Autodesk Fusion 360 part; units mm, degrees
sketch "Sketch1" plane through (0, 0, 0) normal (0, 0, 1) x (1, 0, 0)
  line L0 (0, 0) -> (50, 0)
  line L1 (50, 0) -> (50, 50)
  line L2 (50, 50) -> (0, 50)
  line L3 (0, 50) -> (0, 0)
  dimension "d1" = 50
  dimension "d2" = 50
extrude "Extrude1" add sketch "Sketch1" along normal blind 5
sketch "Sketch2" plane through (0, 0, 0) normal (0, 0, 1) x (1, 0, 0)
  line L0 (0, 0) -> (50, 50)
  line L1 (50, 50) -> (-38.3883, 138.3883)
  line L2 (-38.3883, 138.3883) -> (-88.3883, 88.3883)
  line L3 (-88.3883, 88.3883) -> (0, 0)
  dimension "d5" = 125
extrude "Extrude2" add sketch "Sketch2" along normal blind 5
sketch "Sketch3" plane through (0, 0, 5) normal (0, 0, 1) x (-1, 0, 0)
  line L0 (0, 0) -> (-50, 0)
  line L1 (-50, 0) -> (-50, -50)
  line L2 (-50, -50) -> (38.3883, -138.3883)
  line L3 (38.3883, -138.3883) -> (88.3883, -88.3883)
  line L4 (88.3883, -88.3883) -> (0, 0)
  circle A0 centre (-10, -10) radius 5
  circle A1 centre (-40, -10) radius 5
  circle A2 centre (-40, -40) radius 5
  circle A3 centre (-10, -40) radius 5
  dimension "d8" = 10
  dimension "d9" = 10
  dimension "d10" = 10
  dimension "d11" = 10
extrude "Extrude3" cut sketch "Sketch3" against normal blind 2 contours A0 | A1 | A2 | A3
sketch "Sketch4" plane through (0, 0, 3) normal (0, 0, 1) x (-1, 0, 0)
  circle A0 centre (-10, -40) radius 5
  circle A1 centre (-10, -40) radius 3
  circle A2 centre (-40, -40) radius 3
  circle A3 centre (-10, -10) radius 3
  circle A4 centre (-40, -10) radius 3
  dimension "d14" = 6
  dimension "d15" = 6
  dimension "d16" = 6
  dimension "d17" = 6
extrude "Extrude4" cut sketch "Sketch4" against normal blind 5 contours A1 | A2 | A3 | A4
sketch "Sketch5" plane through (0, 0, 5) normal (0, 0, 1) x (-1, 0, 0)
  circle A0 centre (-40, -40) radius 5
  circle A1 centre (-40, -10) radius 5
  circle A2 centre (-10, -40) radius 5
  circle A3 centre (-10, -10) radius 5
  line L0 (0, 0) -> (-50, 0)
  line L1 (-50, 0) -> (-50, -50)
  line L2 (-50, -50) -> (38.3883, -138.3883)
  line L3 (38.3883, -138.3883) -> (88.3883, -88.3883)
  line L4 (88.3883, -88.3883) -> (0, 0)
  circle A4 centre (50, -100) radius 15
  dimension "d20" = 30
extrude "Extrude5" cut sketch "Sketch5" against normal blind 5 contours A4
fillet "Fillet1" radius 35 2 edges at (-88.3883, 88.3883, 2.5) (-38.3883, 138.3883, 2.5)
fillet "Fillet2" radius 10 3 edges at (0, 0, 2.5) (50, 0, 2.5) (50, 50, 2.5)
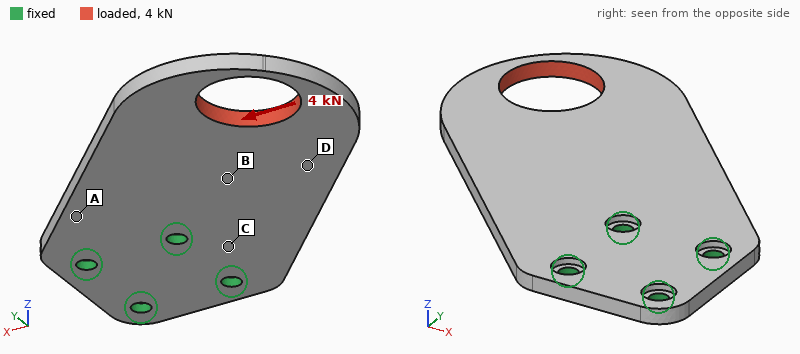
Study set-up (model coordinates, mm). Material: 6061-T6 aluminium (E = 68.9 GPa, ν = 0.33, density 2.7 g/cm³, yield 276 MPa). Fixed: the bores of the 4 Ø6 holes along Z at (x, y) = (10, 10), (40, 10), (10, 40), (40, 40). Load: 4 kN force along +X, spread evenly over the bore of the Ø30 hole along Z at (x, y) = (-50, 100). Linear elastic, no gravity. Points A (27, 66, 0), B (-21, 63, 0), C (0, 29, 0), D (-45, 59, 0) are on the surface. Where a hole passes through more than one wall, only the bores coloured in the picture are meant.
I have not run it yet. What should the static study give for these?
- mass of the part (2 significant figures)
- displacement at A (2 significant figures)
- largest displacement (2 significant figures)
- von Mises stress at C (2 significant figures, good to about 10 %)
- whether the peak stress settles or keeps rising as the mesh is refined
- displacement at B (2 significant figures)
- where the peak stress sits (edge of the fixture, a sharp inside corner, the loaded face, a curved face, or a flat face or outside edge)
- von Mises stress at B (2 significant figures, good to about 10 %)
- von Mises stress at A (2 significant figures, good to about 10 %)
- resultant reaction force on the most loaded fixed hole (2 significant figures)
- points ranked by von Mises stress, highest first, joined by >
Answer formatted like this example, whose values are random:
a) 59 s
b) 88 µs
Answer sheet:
a) 120 g
b) 0.039 mm
c) 0.23 mm
d) 34 MPa
e) keeps rising
f) 0.064 mm
g) edge of the fixture
h) 23 MPa
i) 53 MPa
j) 4.7 kN
k) A > C > B > D
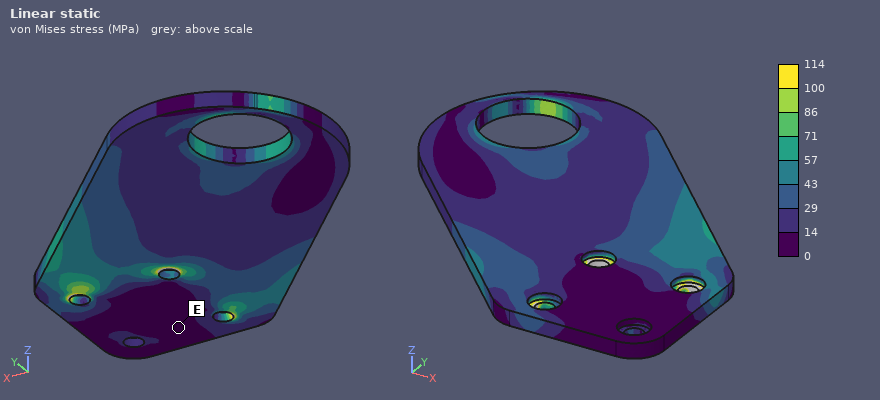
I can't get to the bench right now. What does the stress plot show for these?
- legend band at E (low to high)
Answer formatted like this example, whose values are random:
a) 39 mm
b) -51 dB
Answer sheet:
a) 0 to 14 MPa
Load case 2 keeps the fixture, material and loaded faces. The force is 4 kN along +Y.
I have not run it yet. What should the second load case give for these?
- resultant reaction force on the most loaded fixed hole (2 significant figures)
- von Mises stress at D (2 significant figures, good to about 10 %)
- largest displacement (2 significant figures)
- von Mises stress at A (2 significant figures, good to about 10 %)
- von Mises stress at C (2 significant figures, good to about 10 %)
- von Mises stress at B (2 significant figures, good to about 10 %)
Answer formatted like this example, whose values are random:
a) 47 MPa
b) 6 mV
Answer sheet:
a) 4.7 kN
b) 25 MPa
c) 0.23 mm
d) 41 MPa
e) 44 MPa
f) 24 MPa
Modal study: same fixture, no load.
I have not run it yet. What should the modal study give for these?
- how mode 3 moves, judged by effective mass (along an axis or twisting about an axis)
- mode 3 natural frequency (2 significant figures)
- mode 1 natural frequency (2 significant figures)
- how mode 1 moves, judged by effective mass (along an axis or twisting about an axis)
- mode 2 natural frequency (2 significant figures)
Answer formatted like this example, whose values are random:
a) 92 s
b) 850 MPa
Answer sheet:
a) along Z
b) 2200 Hz
c) 460 Hz
d) along Z
e) 1100 Hz
